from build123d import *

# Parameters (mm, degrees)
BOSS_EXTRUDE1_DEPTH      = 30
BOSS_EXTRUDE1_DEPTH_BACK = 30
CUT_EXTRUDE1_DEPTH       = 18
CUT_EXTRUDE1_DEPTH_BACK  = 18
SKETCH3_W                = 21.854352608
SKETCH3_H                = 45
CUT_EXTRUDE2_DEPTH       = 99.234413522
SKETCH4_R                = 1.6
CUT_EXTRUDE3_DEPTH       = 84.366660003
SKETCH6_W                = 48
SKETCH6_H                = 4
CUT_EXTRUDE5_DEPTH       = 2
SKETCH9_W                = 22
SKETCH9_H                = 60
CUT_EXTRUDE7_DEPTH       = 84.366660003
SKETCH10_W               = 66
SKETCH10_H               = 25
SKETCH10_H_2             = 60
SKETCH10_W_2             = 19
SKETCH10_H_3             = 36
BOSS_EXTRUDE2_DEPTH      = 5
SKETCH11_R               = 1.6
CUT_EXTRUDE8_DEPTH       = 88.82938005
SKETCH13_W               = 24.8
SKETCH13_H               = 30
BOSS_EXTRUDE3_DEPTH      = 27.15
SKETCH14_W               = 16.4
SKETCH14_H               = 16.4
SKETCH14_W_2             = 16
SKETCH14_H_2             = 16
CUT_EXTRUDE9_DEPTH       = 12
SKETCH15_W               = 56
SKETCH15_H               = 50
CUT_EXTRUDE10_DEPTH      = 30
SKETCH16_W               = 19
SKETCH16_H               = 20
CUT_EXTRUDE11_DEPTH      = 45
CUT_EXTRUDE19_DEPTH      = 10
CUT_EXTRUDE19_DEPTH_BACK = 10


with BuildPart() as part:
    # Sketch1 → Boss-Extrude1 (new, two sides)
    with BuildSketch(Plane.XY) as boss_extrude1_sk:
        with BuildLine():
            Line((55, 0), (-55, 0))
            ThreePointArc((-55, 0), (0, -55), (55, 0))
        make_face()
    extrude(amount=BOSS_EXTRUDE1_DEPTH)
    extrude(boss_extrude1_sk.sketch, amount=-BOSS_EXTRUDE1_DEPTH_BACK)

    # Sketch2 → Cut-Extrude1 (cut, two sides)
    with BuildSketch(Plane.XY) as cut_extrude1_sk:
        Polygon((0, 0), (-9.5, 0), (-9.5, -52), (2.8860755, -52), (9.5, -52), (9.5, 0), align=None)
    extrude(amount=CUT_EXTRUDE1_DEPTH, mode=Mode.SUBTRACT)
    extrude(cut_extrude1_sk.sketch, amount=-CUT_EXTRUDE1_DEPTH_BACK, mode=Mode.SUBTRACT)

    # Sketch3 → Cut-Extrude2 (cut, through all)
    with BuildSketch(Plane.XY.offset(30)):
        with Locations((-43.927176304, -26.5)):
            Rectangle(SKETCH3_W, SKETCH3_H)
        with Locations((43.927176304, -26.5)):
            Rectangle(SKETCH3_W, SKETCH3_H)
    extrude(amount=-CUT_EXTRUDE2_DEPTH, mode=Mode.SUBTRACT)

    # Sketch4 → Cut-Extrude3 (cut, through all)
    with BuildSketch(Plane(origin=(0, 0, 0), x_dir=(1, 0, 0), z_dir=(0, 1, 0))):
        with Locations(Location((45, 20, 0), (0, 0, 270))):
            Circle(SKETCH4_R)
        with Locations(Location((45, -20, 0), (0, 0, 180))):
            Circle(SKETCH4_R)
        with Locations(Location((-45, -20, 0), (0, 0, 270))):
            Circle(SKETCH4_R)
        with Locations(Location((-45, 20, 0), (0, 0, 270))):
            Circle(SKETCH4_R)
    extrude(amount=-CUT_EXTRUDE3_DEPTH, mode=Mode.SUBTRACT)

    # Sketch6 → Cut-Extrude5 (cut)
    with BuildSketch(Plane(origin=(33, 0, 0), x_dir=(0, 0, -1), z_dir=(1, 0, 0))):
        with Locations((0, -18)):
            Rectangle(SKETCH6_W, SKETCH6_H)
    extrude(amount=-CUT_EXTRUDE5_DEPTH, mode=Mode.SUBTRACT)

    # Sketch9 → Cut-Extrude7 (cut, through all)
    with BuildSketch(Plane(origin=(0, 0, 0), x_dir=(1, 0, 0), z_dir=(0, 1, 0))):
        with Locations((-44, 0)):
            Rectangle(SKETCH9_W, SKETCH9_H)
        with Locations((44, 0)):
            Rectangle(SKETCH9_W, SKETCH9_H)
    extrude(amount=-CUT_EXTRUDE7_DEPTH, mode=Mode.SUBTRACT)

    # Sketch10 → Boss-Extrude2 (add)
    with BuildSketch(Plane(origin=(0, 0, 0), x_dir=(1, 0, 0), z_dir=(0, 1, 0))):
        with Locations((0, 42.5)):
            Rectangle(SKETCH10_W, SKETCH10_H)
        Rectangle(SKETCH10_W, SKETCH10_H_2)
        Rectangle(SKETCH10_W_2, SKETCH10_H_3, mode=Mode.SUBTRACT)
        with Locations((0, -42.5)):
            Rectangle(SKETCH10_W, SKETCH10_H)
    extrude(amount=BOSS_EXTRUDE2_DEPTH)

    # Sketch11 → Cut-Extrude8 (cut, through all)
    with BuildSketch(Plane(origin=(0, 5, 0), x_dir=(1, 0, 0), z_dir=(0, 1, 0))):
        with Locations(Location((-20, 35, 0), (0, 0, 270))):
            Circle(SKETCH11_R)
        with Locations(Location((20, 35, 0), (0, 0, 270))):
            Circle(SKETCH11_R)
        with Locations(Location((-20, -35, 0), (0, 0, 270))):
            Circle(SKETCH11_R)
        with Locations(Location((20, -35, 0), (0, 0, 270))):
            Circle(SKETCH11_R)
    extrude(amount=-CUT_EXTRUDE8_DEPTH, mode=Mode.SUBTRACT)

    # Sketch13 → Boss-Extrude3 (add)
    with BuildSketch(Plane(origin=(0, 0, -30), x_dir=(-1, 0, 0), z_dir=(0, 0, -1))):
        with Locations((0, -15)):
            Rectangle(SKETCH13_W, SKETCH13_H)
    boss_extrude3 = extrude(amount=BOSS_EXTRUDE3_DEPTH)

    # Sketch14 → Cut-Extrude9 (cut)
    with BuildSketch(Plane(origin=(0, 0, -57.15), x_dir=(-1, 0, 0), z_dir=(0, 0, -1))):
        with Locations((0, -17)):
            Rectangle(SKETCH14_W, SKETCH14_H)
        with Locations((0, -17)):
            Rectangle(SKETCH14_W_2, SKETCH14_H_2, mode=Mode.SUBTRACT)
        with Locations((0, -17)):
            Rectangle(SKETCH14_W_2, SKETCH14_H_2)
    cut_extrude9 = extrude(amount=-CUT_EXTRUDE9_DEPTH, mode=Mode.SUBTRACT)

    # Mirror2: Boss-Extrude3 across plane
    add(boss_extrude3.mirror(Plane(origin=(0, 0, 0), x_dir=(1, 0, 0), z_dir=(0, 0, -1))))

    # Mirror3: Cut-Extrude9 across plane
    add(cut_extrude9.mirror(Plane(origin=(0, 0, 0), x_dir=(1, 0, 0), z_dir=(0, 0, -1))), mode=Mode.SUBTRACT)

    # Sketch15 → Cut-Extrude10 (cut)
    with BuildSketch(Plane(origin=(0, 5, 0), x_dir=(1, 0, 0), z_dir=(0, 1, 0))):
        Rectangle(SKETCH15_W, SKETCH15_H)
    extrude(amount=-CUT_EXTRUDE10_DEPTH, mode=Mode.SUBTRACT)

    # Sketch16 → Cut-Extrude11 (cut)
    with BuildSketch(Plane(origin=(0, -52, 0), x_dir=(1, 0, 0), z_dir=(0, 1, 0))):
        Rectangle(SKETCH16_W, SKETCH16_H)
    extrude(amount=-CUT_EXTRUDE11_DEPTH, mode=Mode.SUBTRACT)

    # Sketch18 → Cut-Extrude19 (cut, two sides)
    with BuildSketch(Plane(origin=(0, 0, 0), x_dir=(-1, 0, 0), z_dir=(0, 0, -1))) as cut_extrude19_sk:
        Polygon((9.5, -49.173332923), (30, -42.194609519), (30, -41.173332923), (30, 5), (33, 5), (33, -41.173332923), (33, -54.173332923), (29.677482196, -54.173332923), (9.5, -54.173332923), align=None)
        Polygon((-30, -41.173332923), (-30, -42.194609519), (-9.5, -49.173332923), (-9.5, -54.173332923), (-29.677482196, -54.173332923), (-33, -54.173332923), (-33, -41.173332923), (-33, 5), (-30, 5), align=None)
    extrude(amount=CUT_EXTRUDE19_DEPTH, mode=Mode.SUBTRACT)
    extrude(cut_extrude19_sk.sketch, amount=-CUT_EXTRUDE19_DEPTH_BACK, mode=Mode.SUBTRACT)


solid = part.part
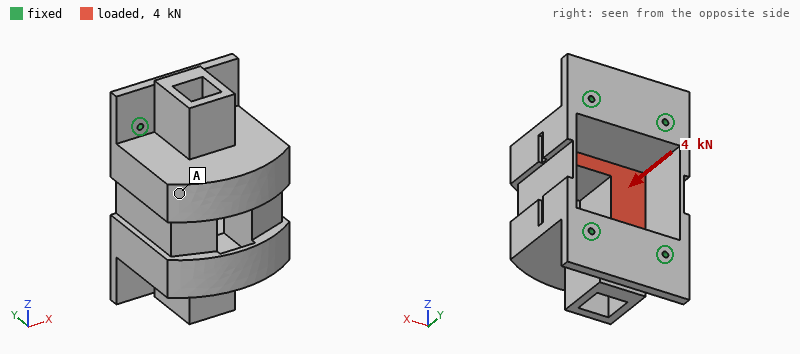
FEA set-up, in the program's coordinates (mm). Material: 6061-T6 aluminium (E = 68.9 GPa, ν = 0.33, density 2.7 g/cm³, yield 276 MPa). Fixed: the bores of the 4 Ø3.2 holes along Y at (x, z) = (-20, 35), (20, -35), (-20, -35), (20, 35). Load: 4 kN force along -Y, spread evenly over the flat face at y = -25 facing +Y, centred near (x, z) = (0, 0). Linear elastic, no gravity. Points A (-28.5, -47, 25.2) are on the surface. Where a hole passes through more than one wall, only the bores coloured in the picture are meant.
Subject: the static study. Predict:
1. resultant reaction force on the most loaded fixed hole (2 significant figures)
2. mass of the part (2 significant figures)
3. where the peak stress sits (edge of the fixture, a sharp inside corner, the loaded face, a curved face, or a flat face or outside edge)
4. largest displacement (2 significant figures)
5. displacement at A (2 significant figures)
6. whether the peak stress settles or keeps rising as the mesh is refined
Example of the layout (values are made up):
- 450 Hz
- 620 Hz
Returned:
- 1.1 kN
- 430 g
- edge of the fixture
- 10 µm
- 7.3 µm
- keeps rising
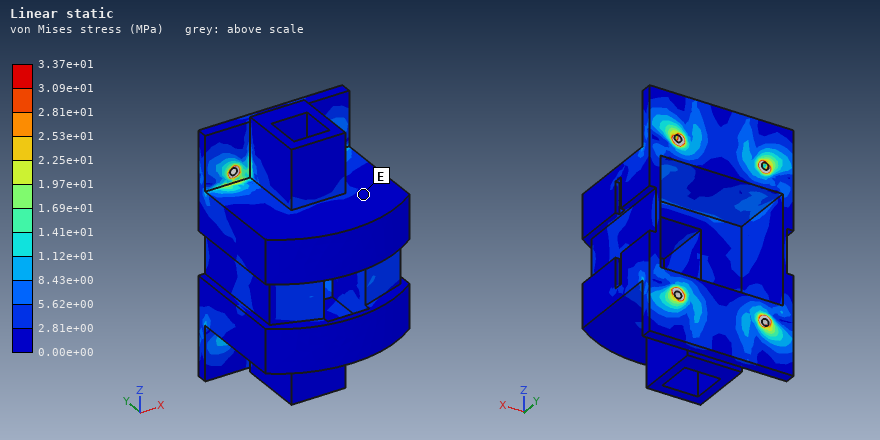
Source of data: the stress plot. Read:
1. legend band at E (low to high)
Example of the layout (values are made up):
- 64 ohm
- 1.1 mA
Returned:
- 0.00e+00 to 2.81e+00 MPa
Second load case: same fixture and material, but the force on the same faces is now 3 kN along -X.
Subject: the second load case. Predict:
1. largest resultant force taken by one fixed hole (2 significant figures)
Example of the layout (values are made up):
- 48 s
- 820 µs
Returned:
- 1.3 kN
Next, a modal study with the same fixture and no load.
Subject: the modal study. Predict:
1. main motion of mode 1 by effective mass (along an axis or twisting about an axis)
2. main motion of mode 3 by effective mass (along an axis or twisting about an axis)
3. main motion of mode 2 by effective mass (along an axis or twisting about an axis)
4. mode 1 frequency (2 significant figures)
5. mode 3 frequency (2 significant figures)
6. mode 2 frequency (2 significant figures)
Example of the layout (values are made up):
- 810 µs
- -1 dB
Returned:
- along X
- along Y
- along Z
- 3200 Hz
- 6100 Hz
- 4000 Hz
